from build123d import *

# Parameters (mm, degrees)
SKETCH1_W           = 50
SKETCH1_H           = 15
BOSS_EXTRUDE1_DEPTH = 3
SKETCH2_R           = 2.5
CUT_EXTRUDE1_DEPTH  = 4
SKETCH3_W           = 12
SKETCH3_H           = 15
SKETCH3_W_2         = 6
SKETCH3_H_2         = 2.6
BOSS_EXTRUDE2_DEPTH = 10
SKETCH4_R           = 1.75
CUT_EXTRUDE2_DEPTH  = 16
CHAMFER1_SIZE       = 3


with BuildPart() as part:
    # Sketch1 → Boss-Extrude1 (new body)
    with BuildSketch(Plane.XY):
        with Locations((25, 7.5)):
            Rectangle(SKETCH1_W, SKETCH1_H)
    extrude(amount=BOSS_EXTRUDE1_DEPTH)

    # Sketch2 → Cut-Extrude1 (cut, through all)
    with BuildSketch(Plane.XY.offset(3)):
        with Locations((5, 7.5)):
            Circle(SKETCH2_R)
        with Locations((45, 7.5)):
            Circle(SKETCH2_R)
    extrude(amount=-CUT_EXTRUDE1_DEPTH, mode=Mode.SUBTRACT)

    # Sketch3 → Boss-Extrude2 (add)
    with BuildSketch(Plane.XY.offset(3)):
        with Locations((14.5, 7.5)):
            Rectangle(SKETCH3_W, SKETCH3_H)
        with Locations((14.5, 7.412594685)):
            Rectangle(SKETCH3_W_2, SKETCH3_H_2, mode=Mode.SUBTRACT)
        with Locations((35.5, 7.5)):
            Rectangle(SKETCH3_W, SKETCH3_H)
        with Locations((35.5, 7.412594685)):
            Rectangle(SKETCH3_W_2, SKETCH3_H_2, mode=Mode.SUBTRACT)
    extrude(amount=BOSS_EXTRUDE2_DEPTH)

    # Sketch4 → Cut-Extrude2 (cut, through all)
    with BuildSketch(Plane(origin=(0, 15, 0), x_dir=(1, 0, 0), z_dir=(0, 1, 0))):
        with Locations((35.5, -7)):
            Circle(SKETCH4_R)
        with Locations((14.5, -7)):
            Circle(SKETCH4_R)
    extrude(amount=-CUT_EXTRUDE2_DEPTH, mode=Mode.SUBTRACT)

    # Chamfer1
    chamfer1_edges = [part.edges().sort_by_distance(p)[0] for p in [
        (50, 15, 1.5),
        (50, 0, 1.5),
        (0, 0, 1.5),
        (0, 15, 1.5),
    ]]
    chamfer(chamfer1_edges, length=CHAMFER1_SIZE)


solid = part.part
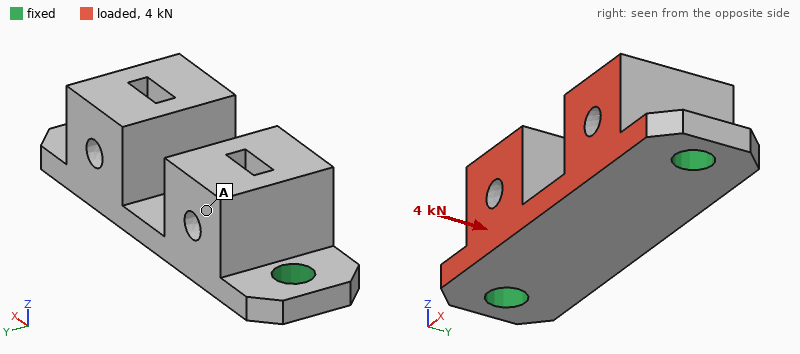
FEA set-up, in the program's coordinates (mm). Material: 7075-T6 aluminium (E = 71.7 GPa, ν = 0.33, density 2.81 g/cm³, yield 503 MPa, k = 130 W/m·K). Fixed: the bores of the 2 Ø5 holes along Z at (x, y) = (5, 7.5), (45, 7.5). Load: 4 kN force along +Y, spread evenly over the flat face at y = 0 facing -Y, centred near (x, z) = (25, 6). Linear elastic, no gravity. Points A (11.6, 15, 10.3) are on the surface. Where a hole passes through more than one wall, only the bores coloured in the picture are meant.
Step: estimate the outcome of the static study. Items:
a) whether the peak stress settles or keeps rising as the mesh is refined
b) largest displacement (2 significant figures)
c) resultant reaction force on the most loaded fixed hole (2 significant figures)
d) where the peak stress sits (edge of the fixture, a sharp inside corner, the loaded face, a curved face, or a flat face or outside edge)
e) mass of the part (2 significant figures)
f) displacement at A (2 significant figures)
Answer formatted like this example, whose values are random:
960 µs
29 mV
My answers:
keeps rising
95 µm
2.0 kN
edge of the fixture
14 g
69 µm
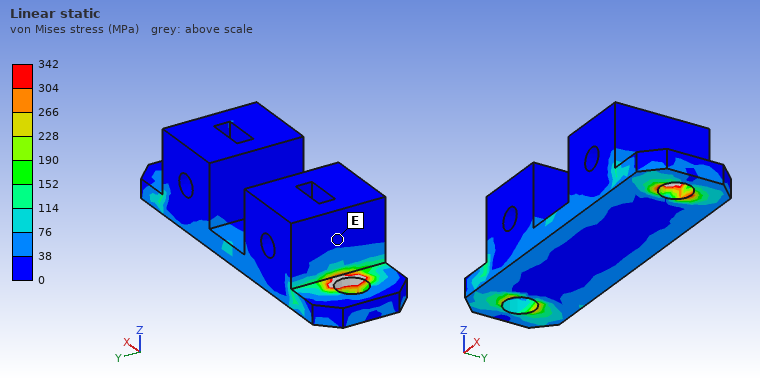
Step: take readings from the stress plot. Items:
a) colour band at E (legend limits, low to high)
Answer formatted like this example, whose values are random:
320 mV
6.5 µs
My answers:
0 to 38 MPa
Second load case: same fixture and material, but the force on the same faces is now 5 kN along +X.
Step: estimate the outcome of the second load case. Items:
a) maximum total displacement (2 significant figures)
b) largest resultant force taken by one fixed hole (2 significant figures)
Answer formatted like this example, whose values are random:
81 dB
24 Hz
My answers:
37 µm
2.7 kN
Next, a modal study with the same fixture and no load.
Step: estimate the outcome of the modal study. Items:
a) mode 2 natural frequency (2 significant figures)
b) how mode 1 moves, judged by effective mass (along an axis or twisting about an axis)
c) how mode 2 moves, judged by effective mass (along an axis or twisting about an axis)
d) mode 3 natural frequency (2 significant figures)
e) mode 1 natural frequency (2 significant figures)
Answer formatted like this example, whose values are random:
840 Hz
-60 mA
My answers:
10 kHz
along Z
along Y
13 kHz
6400 Hz
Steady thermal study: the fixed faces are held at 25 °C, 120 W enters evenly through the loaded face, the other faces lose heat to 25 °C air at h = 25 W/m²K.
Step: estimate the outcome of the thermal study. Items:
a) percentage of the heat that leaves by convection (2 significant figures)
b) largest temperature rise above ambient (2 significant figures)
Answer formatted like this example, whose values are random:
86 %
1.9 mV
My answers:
3.0 %
78 K
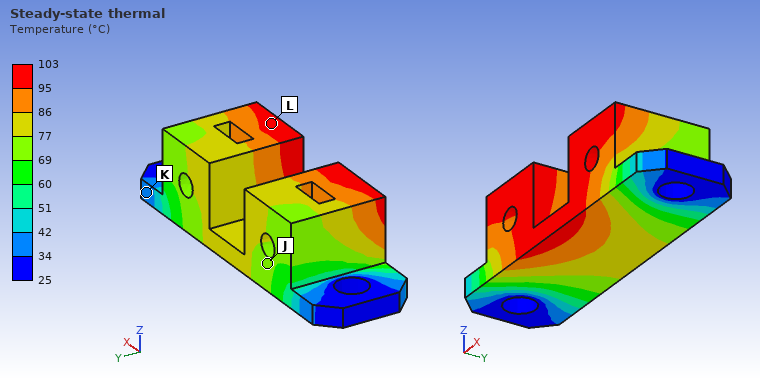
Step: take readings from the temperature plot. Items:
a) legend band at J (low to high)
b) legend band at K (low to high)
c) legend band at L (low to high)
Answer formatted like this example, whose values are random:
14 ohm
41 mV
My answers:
69 to 77 °C
34 to 42 °C
95 to 103 °C
